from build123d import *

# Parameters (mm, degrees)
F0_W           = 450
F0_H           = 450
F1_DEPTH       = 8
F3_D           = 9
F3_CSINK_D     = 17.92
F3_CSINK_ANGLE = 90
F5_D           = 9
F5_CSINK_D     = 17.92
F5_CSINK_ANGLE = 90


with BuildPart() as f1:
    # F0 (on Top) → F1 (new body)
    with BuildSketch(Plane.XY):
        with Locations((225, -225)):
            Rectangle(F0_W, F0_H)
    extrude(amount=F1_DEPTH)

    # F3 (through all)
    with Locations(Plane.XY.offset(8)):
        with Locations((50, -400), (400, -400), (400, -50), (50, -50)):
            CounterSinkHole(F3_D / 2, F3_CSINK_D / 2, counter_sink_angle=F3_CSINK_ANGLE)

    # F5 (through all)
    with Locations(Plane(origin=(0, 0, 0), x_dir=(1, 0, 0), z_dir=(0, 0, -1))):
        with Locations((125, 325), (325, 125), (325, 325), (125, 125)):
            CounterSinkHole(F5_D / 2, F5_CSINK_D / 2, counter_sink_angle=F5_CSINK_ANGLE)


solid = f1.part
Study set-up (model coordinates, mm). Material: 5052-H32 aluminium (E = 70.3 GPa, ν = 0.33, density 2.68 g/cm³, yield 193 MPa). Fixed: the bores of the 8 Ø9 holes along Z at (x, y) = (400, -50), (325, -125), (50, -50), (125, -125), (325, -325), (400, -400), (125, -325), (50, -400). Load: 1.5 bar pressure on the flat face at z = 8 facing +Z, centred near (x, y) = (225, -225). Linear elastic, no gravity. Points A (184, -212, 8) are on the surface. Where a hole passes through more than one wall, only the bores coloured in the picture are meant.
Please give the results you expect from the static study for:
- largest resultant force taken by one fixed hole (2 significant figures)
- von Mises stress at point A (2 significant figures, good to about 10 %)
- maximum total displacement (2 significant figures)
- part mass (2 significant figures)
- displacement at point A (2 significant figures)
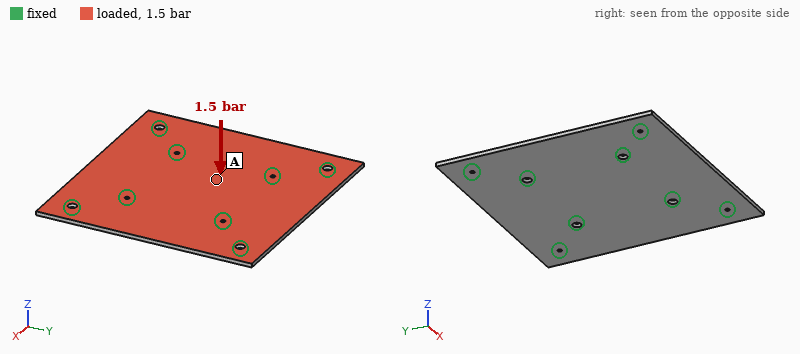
5.4 kN
17 MPa
1.1 mm
4.3 kg
0.40 mm
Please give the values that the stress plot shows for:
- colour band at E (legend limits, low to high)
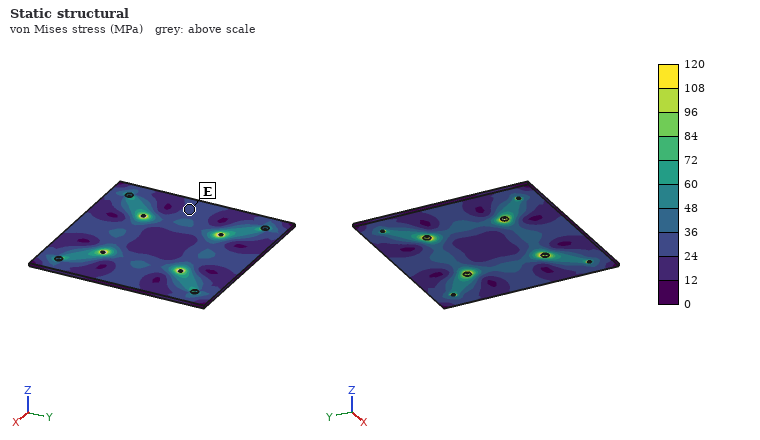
24 to 36 MPa
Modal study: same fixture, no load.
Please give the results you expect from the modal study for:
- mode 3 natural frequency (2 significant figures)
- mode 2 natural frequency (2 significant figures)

450 Hz
450 Hz
